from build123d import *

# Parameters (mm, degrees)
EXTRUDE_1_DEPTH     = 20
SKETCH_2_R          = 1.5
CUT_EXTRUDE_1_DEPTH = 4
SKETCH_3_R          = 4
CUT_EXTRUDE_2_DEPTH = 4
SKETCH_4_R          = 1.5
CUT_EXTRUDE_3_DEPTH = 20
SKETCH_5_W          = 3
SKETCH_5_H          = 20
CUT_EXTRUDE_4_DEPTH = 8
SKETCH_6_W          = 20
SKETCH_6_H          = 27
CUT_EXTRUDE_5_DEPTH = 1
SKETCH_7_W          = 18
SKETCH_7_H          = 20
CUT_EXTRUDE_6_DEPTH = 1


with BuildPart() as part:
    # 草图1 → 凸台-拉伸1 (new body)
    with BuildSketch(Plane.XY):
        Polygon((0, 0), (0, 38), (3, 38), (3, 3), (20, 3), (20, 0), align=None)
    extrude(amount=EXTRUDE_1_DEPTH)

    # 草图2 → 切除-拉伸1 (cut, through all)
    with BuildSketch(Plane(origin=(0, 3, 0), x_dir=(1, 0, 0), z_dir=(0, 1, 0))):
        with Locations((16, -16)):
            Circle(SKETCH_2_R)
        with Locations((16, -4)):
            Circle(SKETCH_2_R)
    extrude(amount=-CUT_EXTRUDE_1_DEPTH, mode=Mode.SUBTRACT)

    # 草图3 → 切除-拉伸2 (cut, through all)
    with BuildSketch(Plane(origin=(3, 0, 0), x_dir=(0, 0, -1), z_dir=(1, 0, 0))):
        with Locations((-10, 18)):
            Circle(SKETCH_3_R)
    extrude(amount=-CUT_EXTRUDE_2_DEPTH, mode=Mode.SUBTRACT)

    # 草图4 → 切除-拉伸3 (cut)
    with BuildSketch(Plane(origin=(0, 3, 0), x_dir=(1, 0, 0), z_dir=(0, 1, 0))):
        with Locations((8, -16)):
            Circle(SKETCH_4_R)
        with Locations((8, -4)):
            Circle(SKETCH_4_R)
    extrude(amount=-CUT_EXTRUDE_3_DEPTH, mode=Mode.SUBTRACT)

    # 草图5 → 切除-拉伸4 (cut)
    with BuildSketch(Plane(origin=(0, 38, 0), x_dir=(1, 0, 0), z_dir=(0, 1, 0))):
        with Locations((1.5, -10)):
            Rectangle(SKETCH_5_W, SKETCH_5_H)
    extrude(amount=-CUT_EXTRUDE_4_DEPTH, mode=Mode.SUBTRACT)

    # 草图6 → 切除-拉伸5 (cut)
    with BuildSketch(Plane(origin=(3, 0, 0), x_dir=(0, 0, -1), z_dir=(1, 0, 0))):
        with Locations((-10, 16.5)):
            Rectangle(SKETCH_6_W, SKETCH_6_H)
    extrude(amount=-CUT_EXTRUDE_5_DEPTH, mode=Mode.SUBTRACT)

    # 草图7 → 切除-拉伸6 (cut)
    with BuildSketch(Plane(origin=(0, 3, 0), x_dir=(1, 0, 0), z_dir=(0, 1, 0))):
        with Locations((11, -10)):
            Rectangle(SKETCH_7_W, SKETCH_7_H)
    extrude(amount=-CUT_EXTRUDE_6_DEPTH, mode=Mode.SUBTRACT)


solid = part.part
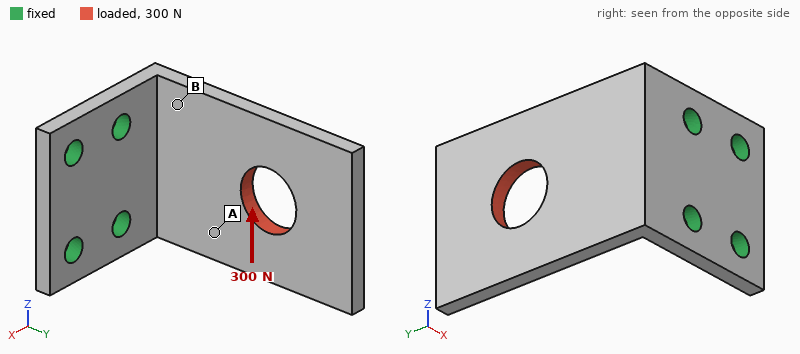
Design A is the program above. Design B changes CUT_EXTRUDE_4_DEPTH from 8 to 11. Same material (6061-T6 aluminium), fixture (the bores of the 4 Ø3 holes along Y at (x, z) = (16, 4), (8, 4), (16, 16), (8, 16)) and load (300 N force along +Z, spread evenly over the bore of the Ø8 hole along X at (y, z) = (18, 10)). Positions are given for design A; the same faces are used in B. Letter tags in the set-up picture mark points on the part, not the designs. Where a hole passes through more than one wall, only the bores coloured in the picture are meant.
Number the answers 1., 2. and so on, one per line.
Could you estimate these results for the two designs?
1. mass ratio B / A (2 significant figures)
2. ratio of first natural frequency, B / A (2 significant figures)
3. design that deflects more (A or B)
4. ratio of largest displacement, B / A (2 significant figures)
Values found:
1. 0.93
2. 1.2
3. A
4. 0.92
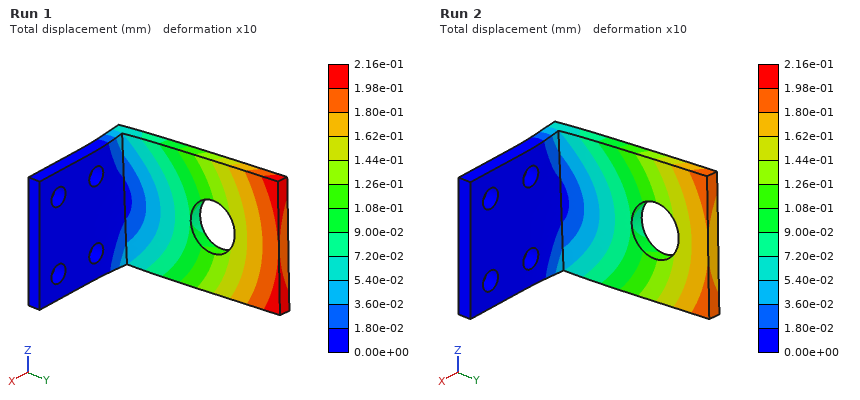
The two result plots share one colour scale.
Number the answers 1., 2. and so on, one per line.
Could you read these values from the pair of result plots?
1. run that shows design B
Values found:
1. Run 2
